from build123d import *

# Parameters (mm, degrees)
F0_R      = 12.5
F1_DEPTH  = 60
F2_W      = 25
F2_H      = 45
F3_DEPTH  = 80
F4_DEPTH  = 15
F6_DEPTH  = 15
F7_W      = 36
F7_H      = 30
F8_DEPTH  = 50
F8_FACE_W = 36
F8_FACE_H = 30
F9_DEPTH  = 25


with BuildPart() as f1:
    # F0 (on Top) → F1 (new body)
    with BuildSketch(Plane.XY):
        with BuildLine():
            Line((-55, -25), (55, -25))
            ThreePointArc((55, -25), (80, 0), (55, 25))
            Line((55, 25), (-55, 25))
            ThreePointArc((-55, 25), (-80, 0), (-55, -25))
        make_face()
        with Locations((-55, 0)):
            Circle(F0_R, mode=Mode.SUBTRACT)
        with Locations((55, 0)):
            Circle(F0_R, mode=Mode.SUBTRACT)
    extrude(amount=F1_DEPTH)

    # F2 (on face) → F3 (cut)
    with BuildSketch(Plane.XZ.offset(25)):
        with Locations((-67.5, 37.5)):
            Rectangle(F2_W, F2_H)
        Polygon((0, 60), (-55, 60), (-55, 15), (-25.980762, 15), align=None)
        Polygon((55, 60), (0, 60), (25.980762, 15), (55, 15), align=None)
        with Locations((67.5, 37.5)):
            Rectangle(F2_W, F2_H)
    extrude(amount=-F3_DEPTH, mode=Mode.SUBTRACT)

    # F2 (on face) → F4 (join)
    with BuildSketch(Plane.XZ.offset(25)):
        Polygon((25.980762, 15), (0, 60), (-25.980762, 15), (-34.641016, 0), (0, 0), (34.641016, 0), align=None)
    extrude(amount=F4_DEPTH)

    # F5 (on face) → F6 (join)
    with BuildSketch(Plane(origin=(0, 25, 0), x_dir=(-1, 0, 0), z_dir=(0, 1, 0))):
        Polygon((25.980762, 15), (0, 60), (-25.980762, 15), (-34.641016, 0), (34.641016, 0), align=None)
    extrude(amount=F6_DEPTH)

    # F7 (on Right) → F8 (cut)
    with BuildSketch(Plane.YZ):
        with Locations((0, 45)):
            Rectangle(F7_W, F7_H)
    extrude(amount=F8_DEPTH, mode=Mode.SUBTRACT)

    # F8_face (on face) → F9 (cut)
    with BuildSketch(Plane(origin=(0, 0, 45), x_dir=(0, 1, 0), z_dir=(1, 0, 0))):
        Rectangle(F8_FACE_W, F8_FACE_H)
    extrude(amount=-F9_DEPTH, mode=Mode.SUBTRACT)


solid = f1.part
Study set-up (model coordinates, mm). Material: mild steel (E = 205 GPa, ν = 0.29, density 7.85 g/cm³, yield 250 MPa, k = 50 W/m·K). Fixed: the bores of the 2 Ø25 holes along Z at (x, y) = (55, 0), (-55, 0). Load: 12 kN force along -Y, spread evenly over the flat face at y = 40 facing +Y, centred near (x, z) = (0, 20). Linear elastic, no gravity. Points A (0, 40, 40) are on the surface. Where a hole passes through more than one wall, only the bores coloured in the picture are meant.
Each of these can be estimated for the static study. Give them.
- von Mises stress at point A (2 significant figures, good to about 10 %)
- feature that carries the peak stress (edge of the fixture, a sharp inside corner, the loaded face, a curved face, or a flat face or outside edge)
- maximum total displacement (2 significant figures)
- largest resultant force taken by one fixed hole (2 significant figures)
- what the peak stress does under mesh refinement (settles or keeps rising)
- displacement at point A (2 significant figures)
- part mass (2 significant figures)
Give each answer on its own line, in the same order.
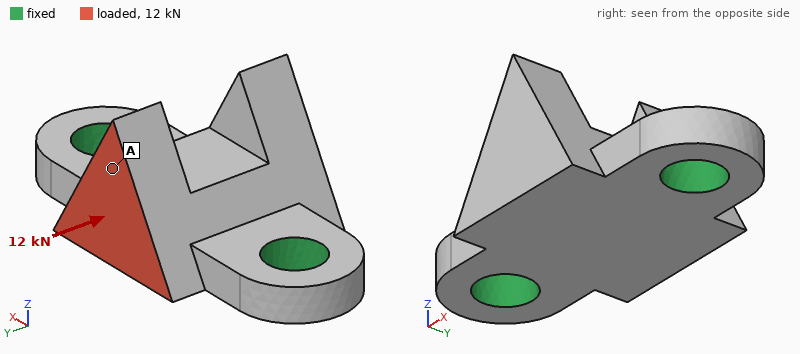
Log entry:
9.2 MPa
edge of the fixture
34 µm
6.0 kN
keeps rising
25 µm
1.6 kg
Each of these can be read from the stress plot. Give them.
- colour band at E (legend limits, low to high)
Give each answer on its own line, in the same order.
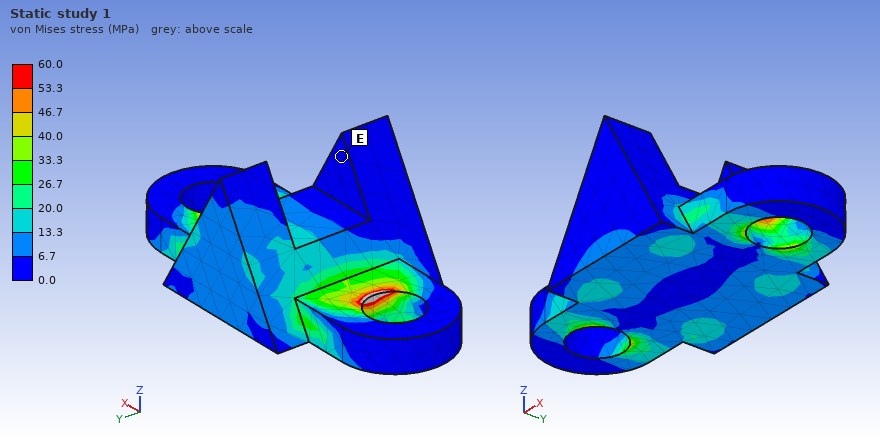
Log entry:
0.0 to 6.7 MPa
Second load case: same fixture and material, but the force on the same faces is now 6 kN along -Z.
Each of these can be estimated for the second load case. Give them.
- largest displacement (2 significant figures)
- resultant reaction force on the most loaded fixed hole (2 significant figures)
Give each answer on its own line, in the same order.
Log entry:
46 µm
3.5 kN
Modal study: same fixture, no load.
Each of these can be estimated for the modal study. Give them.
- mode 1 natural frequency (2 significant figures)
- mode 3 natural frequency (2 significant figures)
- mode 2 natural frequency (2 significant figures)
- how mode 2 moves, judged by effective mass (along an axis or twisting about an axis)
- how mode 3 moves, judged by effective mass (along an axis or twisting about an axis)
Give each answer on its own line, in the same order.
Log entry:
3400 Hz
9300 Hz
5700 Hz
along Z
along X
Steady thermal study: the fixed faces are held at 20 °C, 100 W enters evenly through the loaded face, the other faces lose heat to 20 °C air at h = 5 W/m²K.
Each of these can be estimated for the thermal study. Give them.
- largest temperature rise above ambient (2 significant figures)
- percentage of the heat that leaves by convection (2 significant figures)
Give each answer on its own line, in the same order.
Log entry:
81 K
3.5 %
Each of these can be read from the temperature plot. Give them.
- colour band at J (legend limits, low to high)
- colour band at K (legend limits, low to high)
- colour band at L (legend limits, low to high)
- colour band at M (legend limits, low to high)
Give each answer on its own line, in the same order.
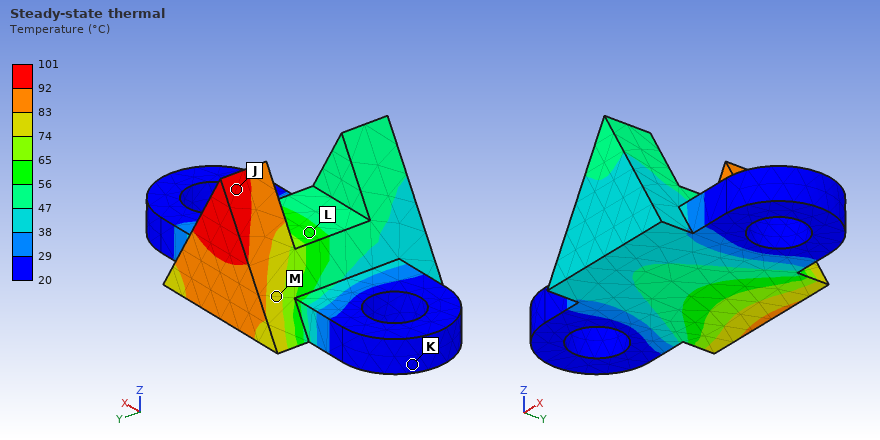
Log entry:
92 to 101 °C
20 to 29 °C
56 to 65 °C
74 to 83 °C
